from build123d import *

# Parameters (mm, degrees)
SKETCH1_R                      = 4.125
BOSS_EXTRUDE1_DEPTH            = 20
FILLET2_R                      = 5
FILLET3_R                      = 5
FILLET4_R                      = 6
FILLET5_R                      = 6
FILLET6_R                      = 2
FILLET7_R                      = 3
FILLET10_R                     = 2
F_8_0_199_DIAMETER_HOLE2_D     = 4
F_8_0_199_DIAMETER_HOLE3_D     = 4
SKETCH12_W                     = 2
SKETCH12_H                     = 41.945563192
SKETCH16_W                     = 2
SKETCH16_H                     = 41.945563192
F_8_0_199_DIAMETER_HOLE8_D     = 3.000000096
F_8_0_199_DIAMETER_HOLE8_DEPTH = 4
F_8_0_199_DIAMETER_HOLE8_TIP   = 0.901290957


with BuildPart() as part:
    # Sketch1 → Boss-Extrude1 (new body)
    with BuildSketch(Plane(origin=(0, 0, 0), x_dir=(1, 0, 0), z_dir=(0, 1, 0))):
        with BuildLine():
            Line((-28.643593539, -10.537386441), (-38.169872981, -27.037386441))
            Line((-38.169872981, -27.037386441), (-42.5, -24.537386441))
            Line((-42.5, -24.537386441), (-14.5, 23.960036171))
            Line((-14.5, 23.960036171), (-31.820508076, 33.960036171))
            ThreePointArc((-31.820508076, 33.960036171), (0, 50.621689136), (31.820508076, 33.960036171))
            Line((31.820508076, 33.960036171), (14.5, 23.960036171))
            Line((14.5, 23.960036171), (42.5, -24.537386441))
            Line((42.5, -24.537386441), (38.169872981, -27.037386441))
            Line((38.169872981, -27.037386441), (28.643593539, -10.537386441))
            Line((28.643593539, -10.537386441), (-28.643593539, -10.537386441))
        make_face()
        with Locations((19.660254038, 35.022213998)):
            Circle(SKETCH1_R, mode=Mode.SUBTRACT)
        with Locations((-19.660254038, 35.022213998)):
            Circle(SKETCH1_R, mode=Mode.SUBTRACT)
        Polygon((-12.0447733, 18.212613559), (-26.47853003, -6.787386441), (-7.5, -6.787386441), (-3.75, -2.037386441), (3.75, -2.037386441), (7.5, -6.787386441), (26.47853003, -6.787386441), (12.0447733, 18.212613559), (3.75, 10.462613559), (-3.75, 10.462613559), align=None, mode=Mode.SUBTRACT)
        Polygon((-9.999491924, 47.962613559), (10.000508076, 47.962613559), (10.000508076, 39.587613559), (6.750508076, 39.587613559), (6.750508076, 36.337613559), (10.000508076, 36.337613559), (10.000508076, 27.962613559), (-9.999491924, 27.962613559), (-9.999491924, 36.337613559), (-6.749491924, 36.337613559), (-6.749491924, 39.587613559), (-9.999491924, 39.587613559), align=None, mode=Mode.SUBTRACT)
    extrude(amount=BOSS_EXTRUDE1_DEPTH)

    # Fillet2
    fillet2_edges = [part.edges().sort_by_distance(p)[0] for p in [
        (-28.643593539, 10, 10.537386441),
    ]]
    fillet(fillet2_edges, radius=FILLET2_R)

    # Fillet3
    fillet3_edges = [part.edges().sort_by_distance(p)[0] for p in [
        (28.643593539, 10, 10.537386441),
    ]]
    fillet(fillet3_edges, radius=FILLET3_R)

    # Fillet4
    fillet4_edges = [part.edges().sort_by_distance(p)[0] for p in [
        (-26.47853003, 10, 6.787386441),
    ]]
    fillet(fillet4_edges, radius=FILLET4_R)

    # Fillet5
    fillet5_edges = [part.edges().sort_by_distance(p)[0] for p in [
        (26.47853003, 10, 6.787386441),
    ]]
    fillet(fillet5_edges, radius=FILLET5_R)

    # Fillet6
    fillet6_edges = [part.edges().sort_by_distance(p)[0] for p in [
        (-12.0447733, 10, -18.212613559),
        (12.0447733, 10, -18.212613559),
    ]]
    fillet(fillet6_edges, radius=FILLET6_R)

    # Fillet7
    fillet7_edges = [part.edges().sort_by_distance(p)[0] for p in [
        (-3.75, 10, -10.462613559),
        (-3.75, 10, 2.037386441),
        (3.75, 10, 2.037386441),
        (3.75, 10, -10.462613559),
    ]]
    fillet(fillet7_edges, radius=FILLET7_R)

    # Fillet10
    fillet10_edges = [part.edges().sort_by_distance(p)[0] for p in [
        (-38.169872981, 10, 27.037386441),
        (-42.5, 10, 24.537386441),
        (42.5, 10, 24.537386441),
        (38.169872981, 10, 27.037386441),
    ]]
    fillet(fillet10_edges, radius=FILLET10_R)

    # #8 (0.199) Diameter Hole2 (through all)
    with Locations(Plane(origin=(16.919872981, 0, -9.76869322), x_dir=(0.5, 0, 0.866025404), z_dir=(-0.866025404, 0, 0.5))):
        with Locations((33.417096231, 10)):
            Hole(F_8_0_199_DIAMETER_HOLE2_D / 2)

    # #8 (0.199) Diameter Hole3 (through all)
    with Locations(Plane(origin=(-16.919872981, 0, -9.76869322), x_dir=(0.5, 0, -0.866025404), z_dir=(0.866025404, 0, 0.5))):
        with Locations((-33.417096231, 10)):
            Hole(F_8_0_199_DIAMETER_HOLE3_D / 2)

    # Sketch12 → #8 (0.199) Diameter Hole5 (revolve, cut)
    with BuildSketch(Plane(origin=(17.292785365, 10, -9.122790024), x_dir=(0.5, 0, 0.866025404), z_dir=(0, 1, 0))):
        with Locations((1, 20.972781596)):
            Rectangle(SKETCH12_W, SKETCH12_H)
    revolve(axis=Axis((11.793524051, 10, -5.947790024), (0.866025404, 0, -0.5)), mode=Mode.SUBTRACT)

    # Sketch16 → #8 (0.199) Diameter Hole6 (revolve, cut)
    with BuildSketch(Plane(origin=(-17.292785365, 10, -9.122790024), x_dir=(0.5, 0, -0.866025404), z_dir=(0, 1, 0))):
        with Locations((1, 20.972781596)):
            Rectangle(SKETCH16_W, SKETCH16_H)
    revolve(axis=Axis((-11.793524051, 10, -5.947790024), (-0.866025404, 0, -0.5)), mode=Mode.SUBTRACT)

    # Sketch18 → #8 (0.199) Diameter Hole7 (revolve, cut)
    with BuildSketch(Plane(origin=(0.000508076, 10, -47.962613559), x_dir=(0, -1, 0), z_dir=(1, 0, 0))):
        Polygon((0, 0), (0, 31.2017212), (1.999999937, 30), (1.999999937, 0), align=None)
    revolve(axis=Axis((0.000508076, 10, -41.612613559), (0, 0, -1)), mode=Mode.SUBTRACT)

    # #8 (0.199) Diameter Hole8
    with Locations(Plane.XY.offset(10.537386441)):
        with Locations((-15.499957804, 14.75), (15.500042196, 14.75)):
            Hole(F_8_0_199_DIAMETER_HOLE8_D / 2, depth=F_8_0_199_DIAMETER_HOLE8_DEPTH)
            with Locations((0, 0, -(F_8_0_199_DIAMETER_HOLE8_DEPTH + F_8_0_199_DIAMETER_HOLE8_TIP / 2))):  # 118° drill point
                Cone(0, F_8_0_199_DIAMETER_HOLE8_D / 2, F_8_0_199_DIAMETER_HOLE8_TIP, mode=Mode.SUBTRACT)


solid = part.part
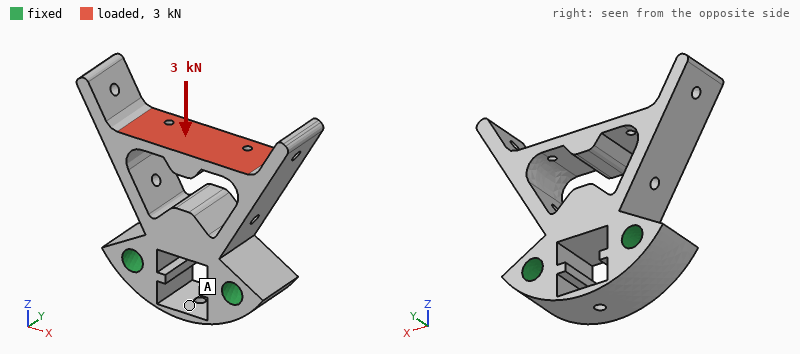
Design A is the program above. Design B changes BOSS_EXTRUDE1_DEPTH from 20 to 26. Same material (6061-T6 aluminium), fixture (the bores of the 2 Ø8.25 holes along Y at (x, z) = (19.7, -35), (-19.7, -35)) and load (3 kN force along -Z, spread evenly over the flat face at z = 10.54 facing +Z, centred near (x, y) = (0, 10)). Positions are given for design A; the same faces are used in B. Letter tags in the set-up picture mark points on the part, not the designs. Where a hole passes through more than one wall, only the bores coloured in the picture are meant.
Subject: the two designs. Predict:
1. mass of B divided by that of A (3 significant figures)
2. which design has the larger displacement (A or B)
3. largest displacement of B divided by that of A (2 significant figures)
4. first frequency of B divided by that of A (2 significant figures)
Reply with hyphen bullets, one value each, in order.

- 1.30
- A
- 0.76
- 1.0
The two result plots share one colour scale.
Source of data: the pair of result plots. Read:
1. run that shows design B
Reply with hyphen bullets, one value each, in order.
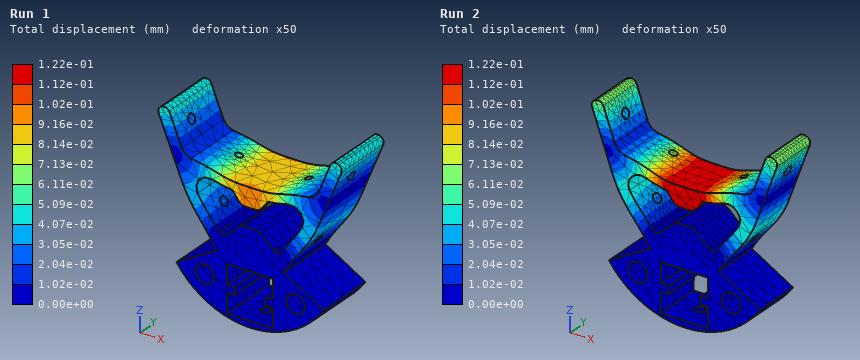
- Run 1
